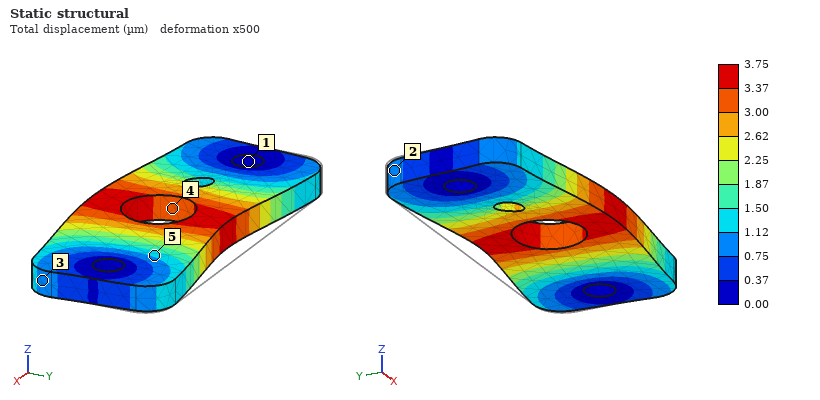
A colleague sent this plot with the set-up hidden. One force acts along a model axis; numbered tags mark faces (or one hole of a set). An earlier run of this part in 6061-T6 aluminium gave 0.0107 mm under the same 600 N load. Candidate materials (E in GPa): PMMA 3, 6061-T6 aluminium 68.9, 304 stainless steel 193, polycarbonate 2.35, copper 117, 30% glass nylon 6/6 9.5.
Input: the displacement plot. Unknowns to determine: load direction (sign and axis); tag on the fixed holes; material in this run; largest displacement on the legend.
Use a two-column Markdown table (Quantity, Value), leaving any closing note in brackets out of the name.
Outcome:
| Quantity | Value |
|---|---|
| load direction | -Y |
| tag on the fixed holes | 1 |
| material in this run | 304 stainless steel |
| largest displacement on the legend | 3.75 µm |
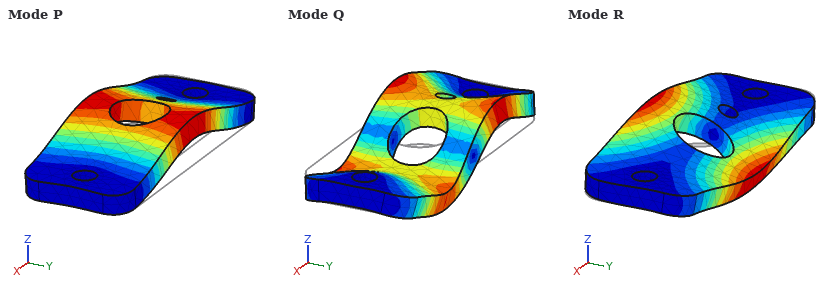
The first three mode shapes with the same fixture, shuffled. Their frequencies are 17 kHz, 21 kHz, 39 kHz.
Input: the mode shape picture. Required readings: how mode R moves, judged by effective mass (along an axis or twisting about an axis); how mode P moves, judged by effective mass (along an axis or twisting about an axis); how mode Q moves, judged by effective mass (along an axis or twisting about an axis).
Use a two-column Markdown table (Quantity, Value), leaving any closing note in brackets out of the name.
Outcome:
| Quantity | Value |
|---|---|
| how mode R moves, judged by effective mass | twisting about X |
| how mode P moves, judged by effective mass | along Z |
| how mode Q moves, judged by effective mass | twisting about Y |
